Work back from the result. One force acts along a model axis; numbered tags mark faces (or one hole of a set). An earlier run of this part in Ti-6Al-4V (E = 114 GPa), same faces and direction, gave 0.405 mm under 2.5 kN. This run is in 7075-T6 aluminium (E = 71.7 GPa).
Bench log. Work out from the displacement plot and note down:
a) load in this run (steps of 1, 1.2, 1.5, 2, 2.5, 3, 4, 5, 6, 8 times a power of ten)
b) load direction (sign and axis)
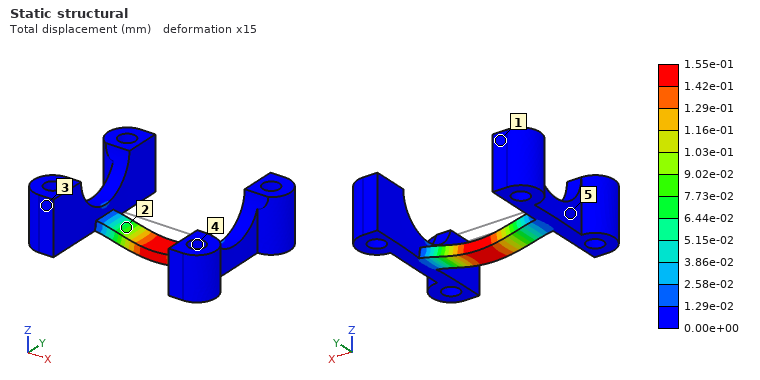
600 N
-Z
